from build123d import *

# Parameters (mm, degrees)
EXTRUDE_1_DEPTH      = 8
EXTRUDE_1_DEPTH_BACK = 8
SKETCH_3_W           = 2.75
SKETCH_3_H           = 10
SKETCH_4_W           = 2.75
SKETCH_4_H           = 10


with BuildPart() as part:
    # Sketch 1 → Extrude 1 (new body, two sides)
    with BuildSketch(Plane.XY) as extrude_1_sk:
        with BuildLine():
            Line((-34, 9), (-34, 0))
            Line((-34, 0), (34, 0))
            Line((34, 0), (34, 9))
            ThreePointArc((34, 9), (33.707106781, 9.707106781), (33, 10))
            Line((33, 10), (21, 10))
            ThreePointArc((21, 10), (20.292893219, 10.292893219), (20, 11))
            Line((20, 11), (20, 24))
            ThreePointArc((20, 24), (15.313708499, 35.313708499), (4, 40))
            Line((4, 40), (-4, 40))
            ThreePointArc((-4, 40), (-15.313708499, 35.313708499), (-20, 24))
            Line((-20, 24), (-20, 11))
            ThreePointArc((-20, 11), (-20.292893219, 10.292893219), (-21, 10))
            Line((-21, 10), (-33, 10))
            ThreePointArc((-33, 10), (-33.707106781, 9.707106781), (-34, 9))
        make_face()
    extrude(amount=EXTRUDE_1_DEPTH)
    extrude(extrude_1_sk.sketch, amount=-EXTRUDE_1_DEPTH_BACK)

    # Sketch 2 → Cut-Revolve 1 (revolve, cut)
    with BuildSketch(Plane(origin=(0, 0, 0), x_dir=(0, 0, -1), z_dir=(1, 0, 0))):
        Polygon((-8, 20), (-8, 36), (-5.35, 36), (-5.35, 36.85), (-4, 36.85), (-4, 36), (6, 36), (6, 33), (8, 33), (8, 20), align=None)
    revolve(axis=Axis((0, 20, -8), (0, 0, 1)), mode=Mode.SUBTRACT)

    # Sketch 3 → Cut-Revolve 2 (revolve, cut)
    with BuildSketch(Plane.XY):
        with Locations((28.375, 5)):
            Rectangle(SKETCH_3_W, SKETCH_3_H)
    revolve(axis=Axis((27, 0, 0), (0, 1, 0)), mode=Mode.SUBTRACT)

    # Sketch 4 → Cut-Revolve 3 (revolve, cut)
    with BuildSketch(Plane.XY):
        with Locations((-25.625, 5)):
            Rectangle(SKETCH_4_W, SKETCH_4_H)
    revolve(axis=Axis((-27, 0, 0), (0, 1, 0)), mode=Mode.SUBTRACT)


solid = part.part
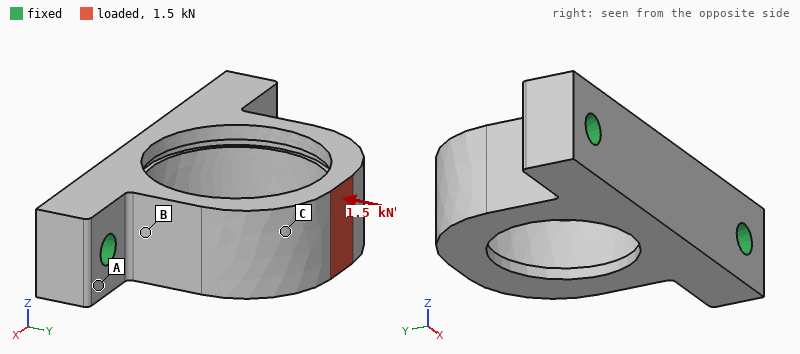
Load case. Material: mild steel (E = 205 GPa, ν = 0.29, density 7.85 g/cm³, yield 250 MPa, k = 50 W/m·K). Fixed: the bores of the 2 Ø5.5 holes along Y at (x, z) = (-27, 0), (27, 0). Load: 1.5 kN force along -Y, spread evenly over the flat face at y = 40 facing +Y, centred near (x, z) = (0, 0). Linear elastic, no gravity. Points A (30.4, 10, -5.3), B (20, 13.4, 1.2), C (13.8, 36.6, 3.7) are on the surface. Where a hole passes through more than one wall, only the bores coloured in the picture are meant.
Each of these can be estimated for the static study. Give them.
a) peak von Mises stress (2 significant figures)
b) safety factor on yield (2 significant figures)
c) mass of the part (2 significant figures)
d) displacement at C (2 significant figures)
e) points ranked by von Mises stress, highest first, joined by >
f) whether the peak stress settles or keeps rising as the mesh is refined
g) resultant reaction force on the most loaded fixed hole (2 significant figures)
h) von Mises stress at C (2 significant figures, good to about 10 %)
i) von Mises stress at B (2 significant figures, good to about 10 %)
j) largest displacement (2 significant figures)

96 MPa
2.6
120 g
3.6 µm
B > C > A
settles
850 N
16 MPa
30 MPa
14 µm
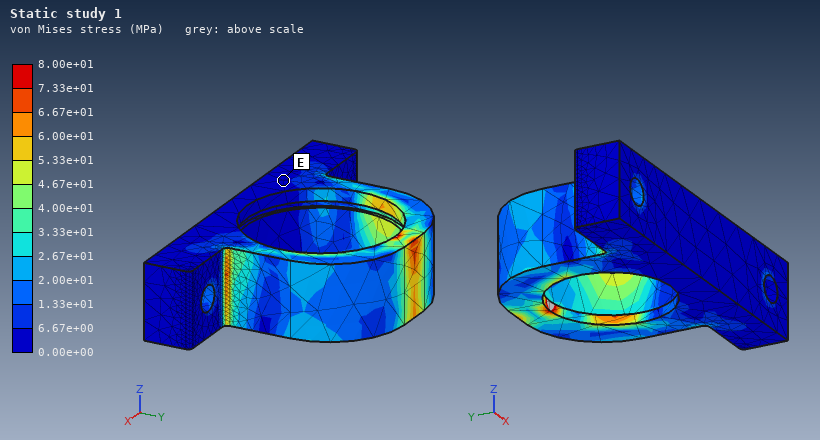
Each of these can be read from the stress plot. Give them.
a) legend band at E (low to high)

0.00e+00 to 6.67e+00 MPa
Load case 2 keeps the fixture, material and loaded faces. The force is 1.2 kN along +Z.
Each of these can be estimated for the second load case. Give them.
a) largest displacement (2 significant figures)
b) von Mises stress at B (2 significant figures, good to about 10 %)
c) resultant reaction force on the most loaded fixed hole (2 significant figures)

55 µm
23 MPa
620 N
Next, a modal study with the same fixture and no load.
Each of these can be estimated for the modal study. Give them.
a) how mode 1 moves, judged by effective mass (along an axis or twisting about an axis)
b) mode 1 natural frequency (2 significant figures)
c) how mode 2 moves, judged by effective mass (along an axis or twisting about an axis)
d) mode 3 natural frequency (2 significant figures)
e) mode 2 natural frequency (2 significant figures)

along Z
5400 Hz
along X
11 kHz
6800 Hz
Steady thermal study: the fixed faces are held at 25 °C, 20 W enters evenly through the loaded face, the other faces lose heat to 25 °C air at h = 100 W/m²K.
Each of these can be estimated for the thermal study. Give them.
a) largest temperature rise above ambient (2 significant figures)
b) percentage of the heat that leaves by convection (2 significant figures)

67 K
59 %
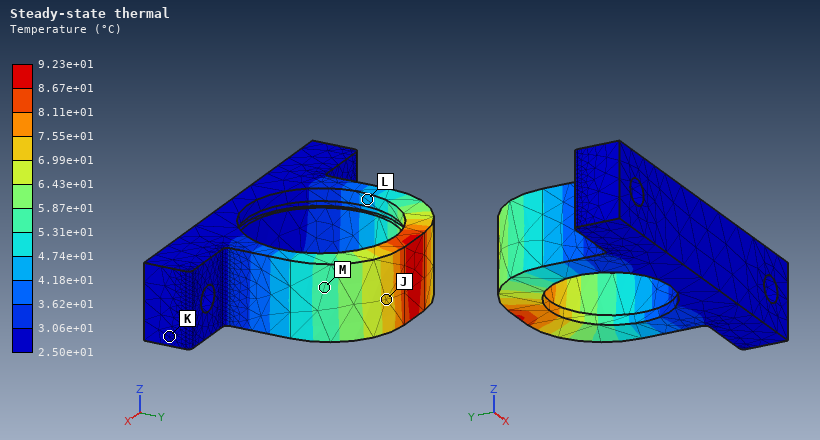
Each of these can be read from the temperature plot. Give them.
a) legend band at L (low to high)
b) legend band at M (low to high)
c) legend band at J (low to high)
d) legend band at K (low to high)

4.18e+01 to 4.74e+01 °C
5.31e+01 to 5.87e+01 °C
6.99e+01 to 7.55e+01 °C
2.50e+01 to 3.06e+01 °C
